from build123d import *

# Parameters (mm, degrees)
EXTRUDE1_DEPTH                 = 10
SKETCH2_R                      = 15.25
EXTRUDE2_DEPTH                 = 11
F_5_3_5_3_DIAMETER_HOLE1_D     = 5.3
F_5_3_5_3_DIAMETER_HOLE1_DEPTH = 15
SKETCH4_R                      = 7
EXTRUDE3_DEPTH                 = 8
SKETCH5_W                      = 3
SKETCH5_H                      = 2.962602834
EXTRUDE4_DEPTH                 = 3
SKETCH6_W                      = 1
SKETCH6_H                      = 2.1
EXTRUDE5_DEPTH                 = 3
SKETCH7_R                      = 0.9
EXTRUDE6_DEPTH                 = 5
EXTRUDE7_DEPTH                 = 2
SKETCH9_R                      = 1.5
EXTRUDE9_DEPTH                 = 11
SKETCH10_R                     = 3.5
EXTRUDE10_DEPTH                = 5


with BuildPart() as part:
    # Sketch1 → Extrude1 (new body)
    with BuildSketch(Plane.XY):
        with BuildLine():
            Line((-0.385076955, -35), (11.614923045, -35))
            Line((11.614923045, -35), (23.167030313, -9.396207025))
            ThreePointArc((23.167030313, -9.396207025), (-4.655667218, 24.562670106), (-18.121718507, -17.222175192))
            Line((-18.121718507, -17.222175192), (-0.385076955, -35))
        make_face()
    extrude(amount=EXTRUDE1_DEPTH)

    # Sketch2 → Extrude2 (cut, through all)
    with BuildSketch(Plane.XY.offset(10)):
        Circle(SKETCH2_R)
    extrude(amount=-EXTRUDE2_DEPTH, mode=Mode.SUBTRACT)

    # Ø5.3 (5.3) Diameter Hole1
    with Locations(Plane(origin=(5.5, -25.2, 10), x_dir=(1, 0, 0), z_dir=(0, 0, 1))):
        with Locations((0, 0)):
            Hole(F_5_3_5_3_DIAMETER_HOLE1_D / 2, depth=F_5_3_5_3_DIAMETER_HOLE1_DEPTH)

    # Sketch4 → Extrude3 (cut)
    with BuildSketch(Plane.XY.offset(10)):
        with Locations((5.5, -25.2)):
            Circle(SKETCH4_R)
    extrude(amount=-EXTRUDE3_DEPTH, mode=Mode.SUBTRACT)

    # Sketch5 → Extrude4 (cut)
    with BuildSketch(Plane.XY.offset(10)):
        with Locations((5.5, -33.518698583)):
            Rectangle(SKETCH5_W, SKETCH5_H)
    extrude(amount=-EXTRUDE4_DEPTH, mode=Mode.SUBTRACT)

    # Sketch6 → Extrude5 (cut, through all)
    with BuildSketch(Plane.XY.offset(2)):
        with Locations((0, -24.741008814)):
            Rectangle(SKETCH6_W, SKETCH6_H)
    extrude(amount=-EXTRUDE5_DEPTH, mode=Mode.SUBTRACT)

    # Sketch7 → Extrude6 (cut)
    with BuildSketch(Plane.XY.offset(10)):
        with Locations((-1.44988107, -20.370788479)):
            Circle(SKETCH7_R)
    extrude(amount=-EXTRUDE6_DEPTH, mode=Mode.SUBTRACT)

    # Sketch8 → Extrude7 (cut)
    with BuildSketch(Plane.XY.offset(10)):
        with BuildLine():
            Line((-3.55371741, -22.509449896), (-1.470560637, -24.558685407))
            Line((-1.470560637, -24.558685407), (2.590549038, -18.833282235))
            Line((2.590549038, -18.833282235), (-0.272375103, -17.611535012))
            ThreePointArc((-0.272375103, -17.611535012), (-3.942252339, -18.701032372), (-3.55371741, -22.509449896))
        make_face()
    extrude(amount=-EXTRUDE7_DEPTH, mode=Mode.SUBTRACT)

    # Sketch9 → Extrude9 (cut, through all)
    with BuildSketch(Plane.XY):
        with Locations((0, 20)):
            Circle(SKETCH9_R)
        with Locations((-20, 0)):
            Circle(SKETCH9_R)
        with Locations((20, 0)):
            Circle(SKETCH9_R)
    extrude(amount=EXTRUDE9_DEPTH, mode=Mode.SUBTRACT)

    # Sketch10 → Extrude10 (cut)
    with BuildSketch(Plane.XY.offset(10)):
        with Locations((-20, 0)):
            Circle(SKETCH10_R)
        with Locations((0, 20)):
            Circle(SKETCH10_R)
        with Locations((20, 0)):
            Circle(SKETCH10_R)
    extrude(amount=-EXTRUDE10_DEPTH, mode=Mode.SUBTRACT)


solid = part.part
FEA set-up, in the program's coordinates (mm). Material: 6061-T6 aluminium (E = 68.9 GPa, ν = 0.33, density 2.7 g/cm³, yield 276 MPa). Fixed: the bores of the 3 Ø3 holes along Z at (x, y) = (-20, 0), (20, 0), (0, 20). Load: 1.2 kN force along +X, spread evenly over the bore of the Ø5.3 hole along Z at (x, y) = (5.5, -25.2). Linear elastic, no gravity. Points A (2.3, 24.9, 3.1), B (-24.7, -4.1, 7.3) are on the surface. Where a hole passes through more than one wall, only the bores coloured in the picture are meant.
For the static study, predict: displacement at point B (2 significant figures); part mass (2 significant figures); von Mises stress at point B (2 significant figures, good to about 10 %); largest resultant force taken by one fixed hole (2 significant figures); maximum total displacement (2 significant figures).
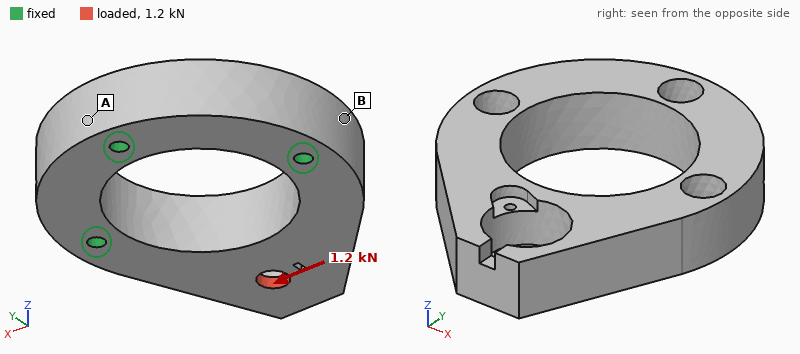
6.1 µm
35 g
16 MPa
910 N
22 µm
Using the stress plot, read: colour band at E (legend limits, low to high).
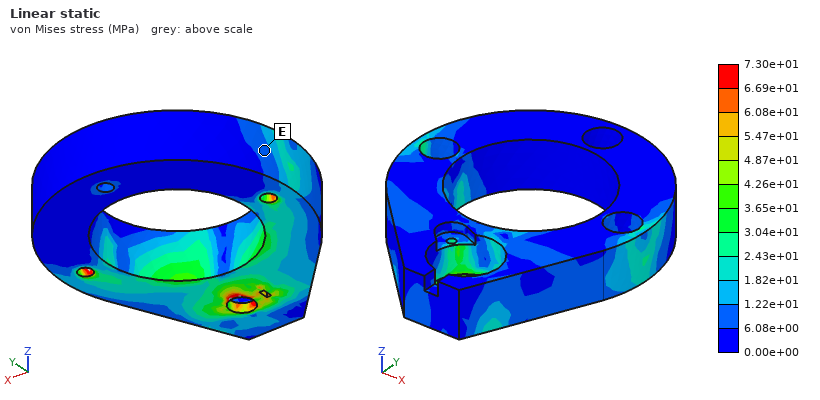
6.08e+00 to 1.22e+01 MPa
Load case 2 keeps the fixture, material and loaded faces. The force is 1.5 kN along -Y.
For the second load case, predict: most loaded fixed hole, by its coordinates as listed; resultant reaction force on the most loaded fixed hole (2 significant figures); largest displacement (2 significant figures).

(20, 0)
1.0 kN
47 µm
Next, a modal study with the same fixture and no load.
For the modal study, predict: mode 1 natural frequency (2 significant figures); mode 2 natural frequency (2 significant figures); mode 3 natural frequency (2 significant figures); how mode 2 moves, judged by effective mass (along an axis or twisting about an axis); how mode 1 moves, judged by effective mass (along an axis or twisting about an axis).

4500 Hz
12 kHz
13 kHz
along X
along Z
